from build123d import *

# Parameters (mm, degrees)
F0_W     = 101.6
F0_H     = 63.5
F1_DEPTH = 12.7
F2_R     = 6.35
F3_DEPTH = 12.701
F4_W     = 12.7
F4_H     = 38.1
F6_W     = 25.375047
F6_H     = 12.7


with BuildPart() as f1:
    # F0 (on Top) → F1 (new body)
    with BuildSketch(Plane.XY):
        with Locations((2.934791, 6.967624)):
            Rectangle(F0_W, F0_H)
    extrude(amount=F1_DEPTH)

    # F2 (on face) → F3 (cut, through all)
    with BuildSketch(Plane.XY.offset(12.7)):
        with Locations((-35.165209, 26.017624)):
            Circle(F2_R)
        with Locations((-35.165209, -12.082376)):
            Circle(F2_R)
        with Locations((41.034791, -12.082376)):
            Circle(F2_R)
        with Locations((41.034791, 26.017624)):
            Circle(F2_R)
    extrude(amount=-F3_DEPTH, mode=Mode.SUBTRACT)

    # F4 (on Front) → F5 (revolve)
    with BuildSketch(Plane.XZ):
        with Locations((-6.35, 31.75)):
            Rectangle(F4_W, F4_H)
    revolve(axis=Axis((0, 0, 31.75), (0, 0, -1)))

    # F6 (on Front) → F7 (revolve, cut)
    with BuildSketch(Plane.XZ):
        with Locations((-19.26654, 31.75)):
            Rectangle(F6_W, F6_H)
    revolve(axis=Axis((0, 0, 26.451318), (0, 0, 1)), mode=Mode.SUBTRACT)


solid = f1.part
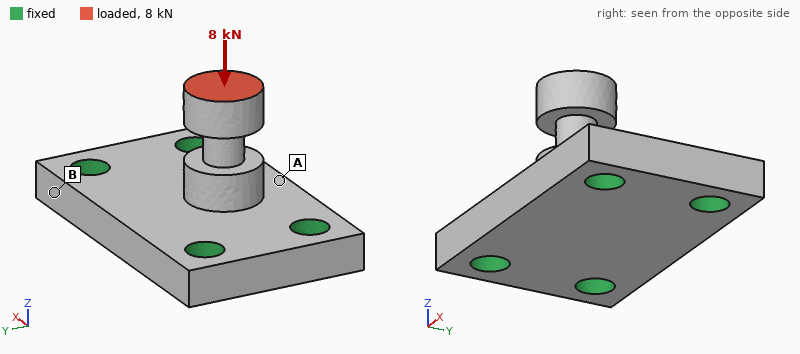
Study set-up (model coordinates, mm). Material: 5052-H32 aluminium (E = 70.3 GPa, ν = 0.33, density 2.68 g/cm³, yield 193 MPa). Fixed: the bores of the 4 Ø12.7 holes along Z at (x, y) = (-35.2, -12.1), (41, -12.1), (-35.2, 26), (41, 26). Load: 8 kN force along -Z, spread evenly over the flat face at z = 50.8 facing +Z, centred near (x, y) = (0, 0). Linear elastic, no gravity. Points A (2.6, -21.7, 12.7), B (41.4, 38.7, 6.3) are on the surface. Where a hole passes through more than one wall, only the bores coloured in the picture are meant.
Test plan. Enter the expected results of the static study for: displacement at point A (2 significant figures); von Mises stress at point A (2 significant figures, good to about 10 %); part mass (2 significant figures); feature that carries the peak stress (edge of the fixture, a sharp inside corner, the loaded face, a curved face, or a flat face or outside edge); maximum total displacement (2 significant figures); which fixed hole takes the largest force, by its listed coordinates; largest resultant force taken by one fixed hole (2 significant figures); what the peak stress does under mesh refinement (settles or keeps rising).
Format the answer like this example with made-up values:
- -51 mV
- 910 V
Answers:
- 22 µm
- 25 MPa
- 240 g
- edge of the fixture
- 46 µm
- (-35.2, -12.1)
- 3.0 kN
- keeps rising
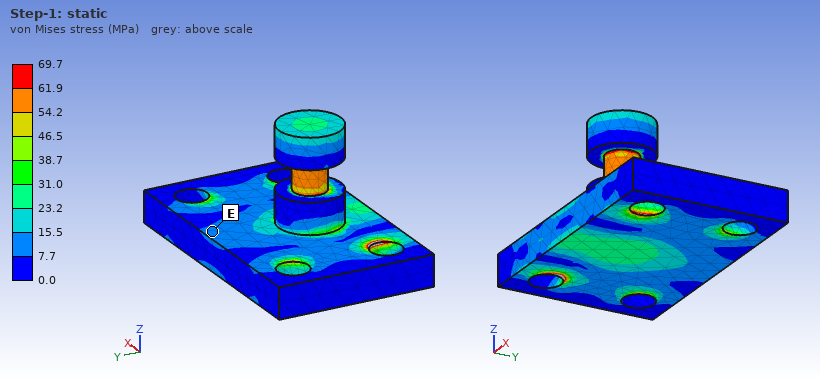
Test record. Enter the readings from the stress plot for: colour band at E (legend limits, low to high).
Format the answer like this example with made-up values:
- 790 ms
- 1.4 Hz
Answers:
- 7.7 to 15.5 MPa
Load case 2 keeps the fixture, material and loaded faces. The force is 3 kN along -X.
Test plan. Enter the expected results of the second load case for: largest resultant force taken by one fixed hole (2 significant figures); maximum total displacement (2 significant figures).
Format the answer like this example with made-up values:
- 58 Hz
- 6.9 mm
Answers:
- 2.0 kN
- 0.31 mm
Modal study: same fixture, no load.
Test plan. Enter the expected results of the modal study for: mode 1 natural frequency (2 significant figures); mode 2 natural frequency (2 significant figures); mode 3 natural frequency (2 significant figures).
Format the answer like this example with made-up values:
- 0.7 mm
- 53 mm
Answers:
- 4600 Hz
- 4900 Hz
- 9000 Hz
